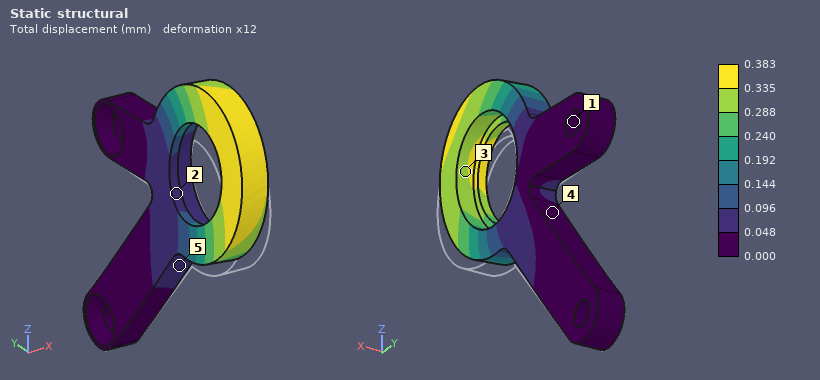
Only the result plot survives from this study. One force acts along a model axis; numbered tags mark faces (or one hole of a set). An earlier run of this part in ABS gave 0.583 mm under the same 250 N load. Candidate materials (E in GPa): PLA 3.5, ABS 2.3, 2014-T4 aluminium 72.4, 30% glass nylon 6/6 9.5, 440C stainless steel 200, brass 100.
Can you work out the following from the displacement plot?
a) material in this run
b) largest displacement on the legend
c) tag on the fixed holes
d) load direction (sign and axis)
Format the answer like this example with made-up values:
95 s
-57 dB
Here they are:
PLA
0.383 mm
1
+Z
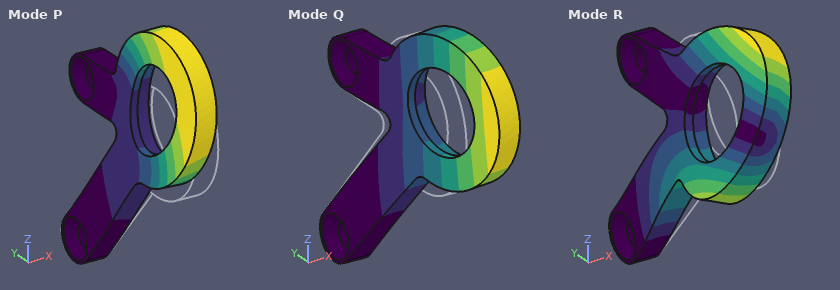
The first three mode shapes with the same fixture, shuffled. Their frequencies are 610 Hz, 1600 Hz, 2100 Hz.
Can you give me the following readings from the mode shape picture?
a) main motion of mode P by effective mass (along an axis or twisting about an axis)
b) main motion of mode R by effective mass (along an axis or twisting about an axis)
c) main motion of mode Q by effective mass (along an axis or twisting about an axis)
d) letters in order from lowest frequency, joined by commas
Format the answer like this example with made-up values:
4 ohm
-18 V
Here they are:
along Z
twisting about Y
along X
Q, R, P
